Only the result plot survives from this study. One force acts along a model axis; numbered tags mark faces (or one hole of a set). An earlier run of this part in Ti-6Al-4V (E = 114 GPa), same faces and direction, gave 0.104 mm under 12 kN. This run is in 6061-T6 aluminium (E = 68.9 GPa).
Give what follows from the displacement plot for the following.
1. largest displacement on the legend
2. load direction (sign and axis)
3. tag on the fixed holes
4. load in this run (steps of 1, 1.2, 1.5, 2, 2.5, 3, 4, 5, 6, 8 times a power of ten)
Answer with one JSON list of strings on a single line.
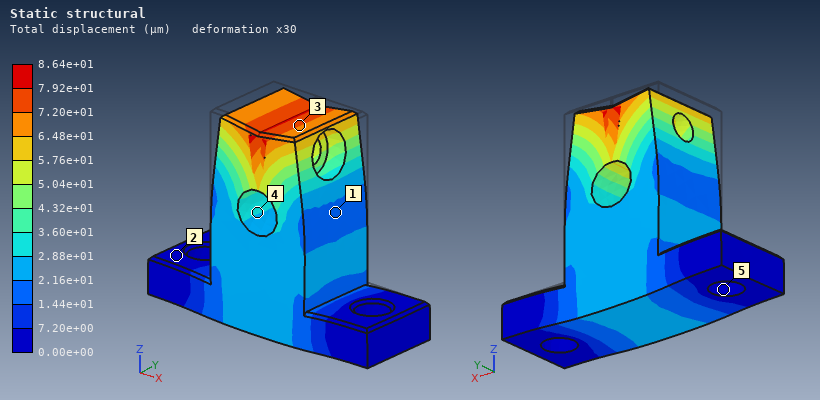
["8.64e+01 µm", "-Z", "5", "6 kN"]
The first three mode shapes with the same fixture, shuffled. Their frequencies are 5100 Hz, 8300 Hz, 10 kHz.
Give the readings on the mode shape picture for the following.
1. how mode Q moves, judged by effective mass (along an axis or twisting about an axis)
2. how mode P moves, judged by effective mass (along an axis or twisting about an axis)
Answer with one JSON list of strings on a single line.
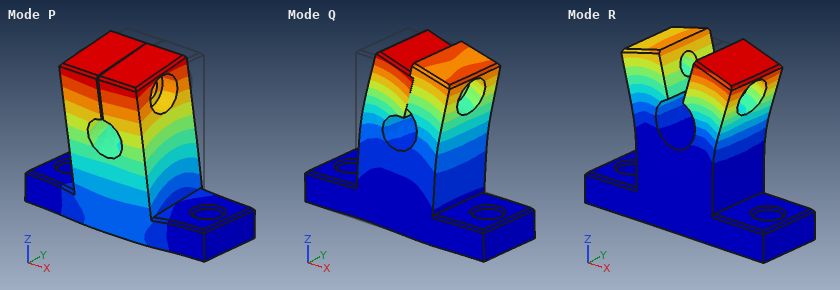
["along X", "along Y"]
